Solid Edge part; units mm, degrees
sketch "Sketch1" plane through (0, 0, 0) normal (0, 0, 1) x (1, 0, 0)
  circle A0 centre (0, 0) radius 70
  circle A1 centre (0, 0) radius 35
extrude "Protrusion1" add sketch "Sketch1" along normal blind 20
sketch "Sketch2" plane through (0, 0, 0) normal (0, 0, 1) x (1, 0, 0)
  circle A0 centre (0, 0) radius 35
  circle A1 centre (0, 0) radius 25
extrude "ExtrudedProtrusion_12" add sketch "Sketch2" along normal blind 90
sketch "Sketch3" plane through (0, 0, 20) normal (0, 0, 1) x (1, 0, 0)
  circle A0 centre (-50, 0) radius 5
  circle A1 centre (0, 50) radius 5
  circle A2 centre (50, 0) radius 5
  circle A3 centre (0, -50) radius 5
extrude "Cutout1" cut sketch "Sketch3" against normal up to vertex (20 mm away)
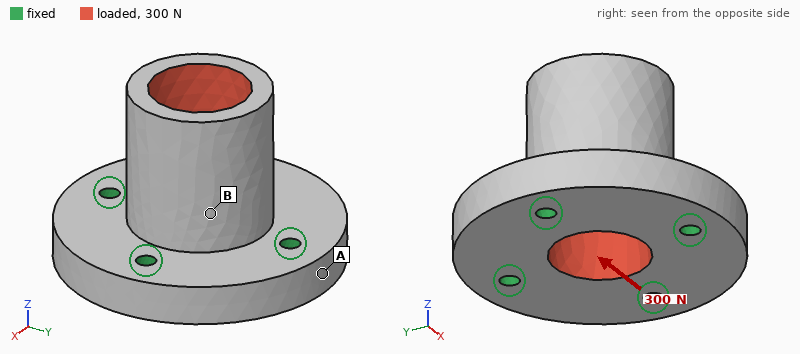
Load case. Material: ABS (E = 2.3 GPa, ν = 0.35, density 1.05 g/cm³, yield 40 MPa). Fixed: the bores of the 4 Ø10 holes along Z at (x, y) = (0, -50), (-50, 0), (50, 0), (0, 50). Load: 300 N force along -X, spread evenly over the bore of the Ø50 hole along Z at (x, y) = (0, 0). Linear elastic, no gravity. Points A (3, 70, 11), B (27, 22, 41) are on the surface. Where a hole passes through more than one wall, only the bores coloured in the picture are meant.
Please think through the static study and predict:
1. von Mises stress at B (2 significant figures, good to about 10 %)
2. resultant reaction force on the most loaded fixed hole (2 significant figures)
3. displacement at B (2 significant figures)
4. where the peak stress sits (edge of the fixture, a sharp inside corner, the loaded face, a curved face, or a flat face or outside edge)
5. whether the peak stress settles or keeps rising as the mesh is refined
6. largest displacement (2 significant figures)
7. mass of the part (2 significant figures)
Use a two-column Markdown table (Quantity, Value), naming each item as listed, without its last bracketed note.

| Quantity | Value |
|---|---|
| von Mises stress at B | 0.16 MPa |
| resultant reaction force on the most loaded fixed hole | 140 N |
| displacement at B | 12 µm |
| where the peak stress sits | edge of the fixture |
| whether the peak stress settles or keeps rising as the mesh is refined | keeps rising |
| largest displacement | 28 µm |
| mass of the part | 410 g |
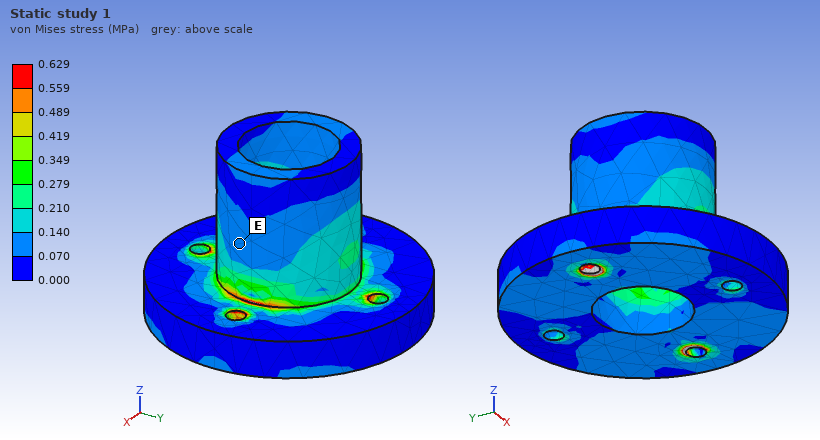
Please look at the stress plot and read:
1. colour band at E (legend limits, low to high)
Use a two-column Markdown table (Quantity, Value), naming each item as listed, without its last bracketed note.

| Quantity | Value |
|---|---|
| colour band at E | 0.070 to 0.140 MPa |
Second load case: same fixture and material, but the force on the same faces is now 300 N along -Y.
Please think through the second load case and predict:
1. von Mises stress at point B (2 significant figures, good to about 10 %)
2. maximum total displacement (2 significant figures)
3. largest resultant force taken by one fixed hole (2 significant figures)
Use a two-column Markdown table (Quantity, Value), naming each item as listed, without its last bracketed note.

| Quantity | Value |
|---|---|
| von Mises stress at point B | 0.19 MPa |
| maximum total displacement | 28 µm |
| largest resultant force taken by one fixed hole | 140 N |
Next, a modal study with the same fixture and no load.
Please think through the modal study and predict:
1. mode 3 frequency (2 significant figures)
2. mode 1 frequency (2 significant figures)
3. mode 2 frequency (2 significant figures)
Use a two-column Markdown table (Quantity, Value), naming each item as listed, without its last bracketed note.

| Quantity | Value |
|---|---|
| mode 3 frequency | 2300 Hz |
| mode 1 frequency | 1400 Hz |
| mode 2 frequency | 1400 Hz |
